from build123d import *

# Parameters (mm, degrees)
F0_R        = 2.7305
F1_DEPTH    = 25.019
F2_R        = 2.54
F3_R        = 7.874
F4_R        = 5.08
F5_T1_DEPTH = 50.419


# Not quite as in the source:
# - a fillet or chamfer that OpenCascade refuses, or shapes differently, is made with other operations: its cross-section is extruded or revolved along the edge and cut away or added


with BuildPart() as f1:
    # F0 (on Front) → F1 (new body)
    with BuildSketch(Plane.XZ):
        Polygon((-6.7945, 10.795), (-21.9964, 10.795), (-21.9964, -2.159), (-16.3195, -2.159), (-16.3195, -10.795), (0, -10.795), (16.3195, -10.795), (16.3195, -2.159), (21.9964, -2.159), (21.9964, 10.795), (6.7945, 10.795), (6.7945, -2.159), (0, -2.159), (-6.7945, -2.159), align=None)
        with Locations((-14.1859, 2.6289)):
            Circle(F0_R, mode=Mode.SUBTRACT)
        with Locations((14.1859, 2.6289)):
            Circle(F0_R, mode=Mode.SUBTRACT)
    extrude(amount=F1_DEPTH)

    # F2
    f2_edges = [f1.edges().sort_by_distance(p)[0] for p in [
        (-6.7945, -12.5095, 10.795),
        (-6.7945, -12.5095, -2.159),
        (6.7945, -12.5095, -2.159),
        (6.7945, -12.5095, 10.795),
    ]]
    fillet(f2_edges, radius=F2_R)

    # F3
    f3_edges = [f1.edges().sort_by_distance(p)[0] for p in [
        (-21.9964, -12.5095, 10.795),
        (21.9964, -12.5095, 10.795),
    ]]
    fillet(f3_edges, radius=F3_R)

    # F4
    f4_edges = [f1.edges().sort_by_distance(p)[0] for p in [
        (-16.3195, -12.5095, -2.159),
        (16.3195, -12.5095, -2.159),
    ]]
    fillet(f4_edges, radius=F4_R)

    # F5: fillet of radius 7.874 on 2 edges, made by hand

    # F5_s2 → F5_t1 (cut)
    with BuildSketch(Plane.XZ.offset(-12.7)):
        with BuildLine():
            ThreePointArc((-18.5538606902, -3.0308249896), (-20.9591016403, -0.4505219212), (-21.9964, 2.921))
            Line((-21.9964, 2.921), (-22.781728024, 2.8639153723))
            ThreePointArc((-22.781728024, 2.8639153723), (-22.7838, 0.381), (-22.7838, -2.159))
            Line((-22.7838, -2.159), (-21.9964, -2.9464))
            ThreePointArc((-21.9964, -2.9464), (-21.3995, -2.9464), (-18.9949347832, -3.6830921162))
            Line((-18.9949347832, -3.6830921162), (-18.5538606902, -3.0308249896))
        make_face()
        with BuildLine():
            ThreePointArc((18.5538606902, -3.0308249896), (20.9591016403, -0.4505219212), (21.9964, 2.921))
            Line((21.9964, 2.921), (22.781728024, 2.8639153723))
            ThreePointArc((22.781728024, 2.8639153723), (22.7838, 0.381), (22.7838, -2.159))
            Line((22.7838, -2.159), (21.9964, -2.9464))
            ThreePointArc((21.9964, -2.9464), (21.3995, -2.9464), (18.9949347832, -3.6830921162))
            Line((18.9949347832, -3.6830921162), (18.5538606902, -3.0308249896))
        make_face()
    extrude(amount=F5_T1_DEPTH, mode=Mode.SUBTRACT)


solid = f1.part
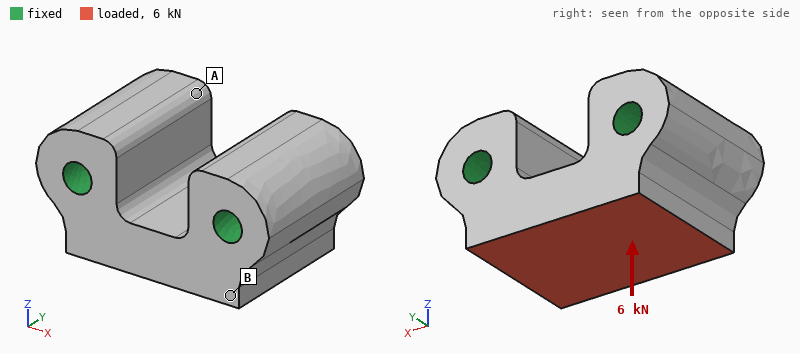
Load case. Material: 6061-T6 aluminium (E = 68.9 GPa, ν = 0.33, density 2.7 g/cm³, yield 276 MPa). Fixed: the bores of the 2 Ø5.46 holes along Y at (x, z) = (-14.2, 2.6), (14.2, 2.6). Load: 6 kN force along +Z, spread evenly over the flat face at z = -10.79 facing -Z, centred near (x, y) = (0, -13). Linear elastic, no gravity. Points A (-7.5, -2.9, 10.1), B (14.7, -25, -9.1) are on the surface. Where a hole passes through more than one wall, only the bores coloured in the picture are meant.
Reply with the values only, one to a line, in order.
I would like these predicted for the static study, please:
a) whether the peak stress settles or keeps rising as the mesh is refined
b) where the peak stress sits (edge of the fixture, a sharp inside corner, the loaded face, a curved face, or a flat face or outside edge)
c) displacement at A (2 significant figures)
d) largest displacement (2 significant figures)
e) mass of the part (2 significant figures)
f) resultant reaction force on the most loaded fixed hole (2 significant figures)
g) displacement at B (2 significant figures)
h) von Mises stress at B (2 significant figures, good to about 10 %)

keeps rising
edge of the fixture
0.90 µm
4.1 µm
41 g
3.3 kN
1.3 µm
7.3 MPa
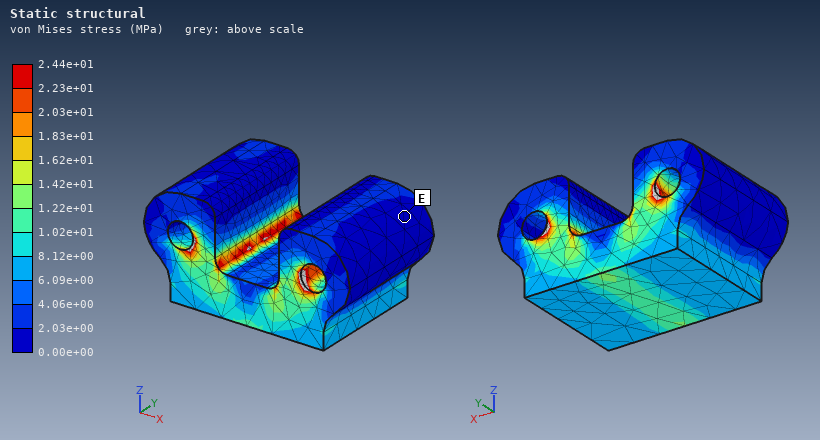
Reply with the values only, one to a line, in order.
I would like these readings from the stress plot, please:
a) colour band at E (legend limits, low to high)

0.00e+00 to 2.03e+00 MPa
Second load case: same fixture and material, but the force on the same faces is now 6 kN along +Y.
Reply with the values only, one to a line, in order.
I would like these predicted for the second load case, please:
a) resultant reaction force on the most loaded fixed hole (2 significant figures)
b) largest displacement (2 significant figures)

3.0 kN
11 µm
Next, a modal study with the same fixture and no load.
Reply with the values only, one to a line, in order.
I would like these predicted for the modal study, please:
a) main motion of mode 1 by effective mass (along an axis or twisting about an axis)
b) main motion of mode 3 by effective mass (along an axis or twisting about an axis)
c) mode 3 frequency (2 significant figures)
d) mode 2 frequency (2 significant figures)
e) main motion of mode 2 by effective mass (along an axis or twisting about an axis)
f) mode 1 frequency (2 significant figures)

along Y
along Z
50 kHz
44 kHz
along X
40 kHz
